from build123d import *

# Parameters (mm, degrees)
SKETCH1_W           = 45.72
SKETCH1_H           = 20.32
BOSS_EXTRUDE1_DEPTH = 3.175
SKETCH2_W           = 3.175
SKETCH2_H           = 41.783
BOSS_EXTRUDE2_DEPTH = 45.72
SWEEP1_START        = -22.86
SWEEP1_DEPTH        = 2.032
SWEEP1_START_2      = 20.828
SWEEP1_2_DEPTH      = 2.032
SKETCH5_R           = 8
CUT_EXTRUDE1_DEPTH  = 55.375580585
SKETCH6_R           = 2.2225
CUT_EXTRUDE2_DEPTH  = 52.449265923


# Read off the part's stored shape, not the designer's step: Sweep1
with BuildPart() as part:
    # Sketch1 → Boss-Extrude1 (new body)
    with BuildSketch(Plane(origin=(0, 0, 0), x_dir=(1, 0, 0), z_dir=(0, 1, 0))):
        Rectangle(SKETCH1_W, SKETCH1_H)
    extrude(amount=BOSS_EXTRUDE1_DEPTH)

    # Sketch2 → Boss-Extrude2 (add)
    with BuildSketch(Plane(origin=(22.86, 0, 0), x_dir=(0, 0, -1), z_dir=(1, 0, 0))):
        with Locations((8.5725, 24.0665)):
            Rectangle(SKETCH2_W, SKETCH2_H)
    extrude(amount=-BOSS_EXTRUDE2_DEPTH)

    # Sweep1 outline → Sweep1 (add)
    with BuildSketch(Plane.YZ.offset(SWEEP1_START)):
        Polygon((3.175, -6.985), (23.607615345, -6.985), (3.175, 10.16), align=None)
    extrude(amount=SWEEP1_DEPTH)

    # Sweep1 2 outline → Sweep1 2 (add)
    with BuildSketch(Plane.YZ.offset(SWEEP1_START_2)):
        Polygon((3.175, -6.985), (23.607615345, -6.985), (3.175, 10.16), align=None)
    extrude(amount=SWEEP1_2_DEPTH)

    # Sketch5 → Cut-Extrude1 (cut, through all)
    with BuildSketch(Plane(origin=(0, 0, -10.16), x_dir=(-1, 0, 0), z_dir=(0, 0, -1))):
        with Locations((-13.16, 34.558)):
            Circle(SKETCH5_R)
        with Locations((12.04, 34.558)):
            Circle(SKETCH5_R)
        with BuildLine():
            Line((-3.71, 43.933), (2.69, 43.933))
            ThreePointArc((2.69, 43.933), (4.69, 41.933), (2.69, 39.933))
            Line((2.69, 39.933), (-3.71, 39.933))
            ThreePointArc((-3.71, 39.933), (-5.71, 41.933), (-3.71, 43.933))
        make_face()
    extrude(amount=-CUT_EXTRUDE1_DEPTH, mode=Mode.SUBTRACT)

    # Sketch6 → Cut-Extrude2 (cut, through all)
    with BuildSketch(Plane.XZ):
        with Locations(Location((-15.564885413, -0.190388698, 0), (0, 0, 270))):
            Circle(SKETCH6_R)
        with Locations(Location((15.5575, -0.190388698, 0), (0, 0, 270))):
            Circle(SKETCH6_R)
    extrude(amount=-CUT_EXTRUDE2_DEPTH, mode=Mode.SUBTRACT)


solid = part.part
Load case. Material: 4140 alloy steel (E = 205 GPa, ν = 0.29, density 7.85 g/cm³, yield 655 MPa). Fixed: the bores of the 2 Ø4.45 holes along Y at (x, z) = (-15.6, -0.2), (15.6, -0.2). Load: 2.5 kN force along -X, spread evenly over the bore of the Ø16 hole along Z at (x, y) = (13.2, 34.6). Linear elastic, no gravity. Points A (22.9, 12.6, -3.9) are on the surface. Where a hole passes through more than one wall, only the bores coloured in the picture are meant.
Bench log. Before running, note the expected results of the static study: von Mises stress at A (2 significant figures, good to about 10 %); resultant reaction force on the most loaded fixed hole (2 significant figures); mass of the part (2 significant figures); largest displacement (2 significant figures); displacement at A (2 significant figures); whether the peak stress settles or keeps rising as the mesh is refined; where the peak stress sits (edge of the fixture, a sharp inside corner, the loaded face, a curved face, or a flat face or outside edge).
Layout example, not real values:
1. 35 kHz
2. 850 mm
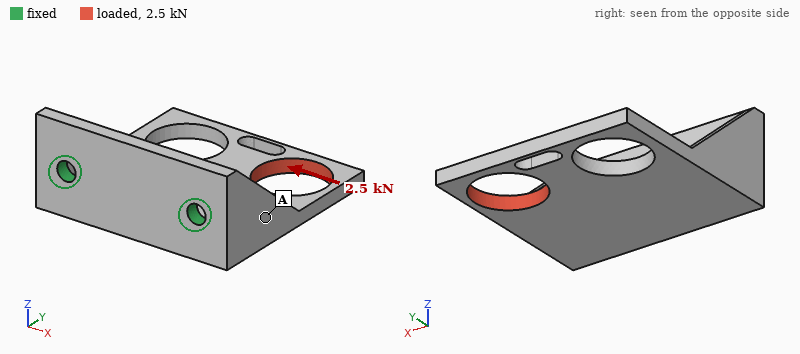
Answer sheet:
1. 70 MPa
2. 2.7 kN
3. 65 g
4. 0.15 mm
5. 0.044 mm
6. keeps rising
7. edge of the fixture
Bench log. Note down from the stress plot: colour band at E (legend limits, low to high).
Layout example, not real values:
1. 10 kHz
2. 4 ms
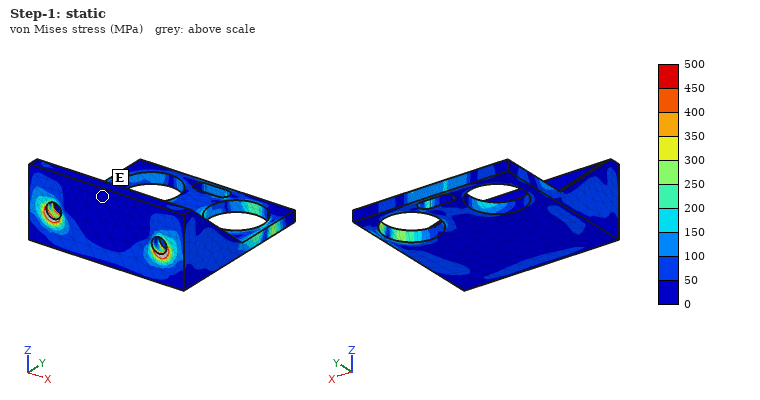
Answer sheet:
1. 0 to 50 MPa
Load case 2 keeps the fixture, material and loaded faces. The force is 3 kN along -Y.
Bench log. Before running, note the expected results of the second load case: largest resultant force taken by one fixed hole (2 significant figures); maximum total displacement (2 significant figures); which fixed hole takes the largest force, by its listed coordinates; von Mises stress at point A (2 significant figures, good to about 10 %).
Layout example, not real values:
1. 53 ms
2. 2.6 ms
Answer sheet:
1. 2.6 kN
2. 0.17 mm
3. (15.6, -0.2)
4. 56 MPa
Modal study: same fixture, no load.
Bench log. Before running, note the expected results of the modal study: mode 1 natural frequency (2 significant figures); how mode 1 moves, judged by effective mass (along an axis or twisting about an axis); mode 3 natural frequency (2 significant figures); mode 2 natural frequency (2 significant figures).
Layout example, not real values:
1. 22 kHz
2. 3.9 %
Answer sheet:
1. 2200 Hz
2. along Z
3. 6700 Hz
4. 4100 Hz
